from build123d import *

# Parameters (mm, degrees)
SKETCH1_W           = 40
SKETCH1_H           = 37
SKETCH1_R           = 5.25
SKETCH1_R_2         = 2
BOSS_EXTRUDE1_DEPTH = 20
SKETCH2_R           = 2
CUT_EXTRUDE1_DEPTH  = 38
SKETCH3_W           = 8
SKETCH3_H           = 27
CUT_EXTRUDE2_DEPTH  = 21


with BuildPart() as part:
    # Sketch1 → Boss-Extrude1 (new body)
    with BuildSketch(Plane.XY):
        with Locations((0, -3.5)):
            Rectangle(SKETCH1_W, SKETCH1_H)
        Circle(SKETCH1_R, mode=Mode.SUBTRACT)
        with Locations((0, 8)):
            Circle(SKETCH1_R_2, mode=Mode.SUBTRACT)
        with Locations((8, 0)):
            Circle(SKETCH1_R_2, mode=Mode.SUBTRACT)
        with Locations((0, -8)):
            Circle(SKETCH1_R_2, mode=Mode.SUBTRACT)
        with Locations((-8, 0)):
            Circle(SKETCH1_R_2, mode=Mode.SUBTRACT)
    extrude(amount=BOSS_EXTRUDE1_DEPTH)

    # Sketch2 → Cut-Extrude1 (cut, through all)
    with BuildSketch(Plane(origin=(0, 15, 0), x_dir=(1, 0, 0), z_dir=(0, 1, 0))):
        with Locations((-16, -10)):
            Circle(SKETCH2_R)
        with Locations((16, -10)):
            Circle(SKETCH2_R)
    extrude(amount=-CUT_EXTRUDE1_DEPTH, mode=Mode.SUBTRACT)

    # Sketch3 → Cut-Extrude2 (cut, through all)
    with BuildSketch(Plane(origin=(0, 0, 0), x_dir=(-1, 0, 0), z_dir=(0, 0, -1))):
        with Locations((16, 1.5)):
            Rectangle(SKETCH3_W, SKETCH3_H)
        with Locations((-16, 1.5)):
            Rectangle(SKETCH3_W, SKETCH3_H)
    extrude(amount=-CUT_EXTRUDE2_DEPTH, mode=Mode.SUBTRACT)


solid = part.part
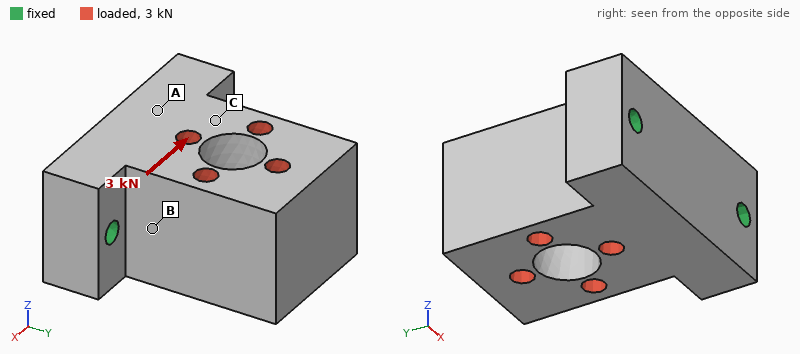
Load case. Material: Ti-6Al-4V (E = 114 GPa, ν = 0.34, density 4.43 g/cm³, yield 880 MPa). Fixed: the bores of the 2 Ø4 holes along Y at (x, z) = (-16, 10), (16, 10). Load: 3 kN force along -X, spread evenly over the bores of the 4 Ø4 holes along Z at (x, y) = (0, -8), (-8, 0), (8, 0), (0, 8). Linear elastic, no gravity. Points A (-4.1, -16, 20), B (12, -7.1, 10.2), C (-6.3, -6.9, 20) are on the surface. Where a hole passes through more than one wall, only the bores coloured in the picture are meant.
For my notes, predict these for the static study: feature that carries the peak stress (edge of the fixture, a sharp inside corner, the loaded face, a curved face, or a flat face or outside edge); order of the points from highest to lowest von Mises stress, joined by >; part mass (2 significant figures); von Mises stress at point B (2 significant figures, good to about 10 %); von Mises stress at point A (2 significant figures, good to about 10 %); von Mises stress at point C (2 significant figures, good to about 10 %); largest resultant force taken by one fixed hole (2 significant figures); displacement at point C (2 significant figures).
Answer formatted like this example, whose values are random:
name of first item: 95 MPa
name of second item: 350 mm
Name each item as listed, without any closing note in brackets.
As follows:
feature that carries the peak stress: the loaded face
order of the points from highest to lowest von Mises stress, joined by >: B > C > A
part mass: 80 g
von Mises stress at point B: 27 MPa
von Mises stress at point A: 7.0 MPa
von Mises stress at point C: 13 MPa
largest resultant force taken by one fixed hole: 2.3 kN
displacement at point C: 3.4 µm
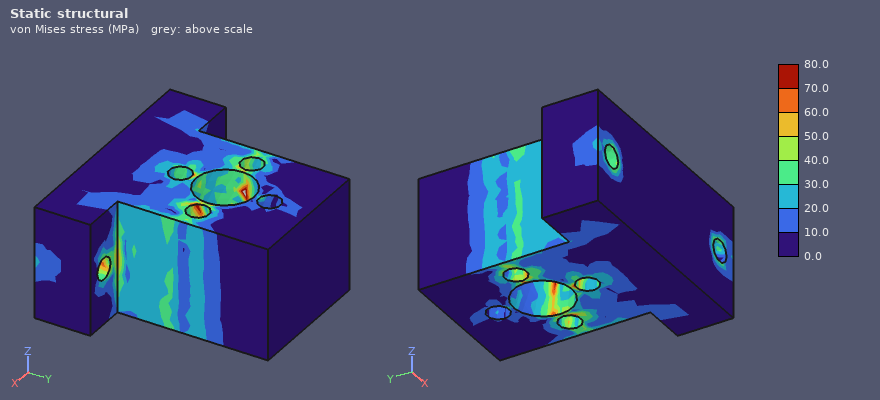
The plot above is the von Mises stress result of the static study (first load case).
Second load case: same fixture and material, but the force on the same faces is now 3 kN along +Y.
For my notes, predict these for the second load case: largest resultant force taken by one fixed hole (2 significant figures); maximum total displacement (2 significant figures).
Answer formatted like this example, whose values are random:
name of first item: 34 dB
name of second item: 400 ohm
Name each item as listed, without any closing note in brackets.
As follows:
largest resultant force taken by one fixed hole: 1.6 kN
maximum total displacement: 4.2 µm
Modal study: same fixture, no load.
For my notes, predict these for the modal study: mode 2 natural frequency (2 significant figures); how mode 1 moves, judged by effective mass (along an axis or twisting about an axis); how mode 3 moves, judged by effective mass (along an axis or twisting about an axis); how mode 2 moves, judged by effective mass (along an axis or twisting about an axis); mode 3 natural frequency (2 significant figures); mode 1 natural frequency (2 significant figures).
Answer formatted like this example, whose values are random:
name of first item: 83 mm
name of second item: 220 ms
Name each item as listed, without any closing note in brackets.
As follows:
mode 2 natural frequency: 10 kHz
how mode 1 moves, judged by effective mass: along Z
how mode 3 moves, judged by effective mass: twisting about Y
how mode 2 moves, judged by effective mass: along X
mode 3 natural frequency: 17 kHz
mode 1 natural frequency: 6400 Hz
